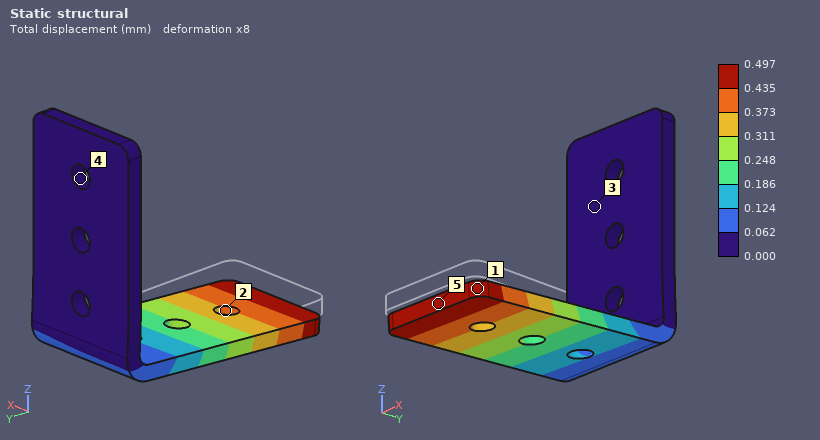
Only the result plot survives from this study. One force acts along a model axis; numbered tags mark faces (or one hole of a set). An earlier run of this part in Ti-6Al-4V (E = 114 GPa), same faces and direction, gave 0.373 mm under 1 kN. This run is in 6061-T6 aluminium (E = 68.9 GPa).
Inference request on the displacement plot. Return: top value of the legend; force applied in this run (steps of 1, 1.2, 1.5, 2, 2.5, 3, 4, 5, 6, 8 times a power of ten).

0.497 mm
800 N
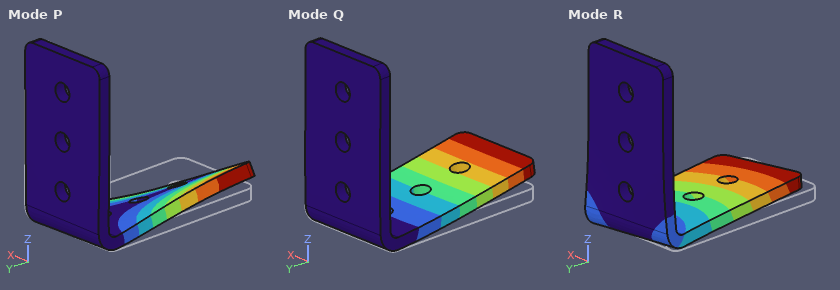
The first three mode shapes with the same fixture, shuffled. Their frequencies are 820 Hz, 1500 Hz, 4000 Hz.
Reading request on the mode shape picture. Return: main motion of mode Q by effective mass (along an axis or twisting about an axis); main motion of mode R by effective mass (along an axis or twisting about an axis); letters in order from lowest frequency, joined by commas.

along Z
along X
Q, R, P
